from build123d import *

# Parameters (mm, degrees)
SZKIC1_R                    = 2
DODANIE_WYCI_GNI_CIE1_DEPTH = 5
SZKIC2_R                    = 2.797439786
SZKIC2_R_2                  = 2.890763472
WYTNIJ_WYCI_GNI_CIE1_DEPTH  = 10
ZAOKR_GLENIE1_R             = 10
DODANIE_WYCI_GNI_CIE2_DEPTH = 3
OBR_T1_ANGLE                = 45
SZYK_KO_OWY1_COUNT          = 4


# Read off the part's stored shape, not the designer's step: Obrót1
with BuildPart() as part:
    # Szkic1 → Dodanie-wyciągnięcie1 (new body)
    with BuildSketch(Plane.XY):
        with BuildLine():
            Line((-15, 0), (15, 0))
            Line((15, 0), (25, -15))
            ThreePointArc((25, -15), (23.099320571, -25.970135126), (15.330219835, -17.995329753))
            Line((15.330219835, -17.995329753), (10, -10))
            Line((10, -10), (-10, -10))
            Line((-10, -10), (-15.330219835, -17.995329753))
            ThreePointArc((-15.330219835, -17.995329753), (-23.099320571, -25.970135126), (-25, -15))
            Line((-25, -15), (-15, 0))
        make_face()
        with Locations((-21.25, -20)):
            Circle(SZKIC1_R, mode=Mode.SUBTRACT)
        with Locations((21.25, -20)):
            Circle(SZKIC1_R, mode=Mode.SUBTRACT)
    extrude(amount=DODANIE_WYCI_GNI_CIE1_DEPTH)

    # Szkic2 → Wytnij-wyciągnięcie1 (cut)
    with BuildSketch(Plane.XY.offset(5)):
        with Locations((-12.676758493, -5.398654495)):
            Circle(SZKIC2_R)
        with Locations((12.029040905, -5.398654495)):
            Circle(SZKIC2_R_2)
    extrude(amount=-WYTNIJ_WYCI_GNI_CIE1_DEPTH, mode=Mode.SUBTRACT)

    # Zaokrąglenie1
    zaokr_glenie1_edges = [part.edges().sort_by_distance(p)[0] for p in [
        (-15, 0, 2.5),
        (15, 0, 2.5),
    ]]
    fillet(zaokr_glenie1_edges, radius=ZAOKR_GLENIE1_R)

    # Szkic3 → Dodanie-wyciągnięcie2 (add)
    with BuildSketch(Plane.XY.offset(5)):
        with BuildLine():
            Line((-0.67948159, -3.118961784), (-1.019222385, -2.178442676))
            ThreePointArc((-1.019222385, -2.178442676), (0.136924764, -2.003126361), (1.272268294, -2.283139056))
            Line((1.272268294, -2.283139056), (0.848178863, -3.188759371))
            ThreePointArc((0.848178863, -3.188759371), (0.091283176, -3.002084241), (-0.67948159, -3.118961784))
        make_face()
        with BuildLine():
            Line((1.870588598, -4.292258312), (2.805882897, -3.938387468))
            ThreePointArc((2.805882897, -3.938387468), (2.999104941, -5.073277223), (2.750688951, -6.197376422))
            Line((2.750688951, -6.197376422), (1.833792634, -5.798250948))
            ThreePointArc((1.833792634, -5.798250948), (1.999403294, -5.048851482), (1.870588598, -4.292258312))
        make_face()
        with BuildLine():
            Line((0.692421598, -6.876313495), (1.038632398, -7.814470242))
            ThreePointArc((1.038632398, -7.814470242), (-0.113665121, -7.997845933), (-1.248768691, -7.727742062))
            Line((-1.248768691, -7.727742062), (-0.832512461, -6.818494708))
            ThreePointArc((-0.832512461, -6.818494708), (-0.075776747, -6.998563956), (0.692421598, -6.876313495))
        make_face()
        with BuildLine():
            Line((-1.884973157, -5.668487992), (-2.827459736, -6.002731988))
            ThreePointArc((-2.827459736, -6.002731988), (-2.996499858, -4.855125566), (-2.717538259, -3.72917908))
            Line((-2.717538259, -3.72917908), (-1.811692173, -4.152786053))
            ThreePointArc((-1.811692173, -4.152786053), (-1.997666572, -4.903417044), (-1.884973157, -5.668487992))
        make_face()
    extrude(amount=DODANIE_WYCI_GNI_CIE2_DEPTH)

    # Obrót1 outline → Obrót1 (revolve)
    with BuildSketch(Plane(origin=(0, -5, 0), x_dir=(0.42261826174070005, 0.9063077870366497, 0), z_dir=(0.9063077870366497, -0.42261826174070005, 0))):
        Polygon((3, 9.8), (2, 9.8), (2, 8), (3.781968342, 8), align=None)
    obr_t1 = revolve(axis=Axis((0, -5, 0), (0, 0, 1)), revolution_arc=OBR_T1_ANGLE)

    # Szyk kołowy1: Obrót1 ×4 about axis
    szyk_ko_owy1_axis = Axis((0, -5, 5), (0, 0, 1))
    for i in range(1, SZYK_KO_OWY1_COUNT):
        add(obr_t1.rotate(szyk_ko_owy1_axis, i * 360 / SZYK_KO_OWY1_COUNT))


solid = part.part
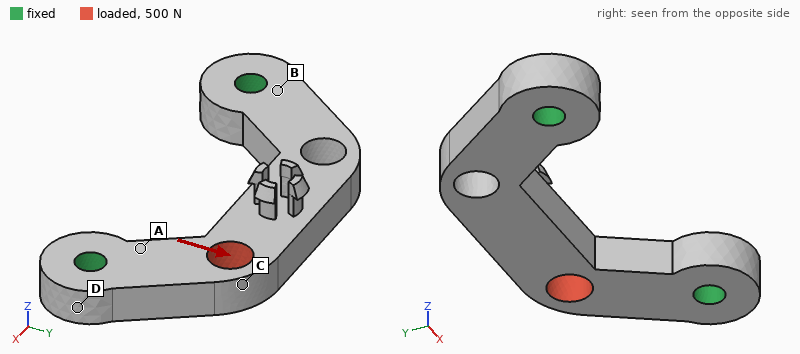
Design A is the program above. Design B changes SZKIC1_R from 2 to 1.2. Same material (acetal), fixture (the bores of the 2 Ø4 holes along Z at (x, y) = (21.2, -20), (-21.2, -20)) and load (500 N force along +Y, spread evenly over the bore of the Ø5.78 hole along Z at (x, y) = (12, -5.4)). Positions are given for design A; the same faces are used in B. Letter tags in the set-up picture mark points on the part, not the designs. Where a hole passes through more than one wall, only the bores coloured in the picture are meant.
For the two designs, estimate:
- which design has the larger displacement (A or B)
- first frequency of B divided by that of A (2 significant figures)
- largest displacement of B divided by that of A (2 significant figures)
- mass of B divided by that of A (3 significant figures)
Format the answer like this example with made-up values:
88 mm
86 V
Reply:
B
0.92
1.1
1.02
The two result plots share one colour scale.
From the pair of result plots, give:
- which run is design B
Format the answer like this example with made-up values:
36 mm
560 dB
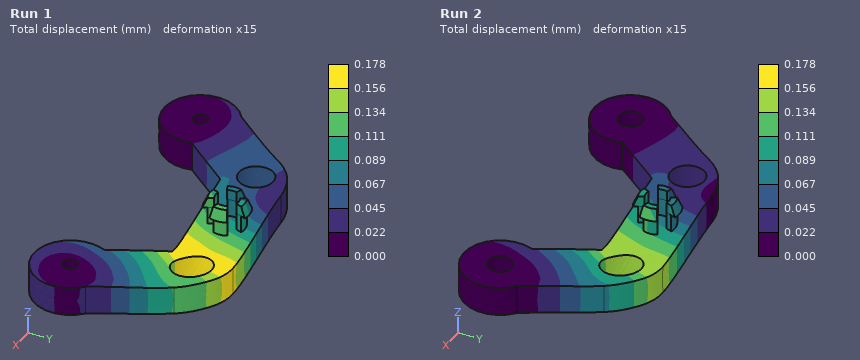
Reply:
Run 1
